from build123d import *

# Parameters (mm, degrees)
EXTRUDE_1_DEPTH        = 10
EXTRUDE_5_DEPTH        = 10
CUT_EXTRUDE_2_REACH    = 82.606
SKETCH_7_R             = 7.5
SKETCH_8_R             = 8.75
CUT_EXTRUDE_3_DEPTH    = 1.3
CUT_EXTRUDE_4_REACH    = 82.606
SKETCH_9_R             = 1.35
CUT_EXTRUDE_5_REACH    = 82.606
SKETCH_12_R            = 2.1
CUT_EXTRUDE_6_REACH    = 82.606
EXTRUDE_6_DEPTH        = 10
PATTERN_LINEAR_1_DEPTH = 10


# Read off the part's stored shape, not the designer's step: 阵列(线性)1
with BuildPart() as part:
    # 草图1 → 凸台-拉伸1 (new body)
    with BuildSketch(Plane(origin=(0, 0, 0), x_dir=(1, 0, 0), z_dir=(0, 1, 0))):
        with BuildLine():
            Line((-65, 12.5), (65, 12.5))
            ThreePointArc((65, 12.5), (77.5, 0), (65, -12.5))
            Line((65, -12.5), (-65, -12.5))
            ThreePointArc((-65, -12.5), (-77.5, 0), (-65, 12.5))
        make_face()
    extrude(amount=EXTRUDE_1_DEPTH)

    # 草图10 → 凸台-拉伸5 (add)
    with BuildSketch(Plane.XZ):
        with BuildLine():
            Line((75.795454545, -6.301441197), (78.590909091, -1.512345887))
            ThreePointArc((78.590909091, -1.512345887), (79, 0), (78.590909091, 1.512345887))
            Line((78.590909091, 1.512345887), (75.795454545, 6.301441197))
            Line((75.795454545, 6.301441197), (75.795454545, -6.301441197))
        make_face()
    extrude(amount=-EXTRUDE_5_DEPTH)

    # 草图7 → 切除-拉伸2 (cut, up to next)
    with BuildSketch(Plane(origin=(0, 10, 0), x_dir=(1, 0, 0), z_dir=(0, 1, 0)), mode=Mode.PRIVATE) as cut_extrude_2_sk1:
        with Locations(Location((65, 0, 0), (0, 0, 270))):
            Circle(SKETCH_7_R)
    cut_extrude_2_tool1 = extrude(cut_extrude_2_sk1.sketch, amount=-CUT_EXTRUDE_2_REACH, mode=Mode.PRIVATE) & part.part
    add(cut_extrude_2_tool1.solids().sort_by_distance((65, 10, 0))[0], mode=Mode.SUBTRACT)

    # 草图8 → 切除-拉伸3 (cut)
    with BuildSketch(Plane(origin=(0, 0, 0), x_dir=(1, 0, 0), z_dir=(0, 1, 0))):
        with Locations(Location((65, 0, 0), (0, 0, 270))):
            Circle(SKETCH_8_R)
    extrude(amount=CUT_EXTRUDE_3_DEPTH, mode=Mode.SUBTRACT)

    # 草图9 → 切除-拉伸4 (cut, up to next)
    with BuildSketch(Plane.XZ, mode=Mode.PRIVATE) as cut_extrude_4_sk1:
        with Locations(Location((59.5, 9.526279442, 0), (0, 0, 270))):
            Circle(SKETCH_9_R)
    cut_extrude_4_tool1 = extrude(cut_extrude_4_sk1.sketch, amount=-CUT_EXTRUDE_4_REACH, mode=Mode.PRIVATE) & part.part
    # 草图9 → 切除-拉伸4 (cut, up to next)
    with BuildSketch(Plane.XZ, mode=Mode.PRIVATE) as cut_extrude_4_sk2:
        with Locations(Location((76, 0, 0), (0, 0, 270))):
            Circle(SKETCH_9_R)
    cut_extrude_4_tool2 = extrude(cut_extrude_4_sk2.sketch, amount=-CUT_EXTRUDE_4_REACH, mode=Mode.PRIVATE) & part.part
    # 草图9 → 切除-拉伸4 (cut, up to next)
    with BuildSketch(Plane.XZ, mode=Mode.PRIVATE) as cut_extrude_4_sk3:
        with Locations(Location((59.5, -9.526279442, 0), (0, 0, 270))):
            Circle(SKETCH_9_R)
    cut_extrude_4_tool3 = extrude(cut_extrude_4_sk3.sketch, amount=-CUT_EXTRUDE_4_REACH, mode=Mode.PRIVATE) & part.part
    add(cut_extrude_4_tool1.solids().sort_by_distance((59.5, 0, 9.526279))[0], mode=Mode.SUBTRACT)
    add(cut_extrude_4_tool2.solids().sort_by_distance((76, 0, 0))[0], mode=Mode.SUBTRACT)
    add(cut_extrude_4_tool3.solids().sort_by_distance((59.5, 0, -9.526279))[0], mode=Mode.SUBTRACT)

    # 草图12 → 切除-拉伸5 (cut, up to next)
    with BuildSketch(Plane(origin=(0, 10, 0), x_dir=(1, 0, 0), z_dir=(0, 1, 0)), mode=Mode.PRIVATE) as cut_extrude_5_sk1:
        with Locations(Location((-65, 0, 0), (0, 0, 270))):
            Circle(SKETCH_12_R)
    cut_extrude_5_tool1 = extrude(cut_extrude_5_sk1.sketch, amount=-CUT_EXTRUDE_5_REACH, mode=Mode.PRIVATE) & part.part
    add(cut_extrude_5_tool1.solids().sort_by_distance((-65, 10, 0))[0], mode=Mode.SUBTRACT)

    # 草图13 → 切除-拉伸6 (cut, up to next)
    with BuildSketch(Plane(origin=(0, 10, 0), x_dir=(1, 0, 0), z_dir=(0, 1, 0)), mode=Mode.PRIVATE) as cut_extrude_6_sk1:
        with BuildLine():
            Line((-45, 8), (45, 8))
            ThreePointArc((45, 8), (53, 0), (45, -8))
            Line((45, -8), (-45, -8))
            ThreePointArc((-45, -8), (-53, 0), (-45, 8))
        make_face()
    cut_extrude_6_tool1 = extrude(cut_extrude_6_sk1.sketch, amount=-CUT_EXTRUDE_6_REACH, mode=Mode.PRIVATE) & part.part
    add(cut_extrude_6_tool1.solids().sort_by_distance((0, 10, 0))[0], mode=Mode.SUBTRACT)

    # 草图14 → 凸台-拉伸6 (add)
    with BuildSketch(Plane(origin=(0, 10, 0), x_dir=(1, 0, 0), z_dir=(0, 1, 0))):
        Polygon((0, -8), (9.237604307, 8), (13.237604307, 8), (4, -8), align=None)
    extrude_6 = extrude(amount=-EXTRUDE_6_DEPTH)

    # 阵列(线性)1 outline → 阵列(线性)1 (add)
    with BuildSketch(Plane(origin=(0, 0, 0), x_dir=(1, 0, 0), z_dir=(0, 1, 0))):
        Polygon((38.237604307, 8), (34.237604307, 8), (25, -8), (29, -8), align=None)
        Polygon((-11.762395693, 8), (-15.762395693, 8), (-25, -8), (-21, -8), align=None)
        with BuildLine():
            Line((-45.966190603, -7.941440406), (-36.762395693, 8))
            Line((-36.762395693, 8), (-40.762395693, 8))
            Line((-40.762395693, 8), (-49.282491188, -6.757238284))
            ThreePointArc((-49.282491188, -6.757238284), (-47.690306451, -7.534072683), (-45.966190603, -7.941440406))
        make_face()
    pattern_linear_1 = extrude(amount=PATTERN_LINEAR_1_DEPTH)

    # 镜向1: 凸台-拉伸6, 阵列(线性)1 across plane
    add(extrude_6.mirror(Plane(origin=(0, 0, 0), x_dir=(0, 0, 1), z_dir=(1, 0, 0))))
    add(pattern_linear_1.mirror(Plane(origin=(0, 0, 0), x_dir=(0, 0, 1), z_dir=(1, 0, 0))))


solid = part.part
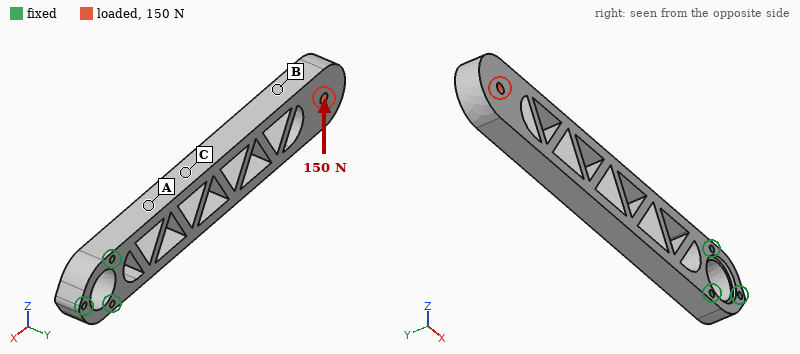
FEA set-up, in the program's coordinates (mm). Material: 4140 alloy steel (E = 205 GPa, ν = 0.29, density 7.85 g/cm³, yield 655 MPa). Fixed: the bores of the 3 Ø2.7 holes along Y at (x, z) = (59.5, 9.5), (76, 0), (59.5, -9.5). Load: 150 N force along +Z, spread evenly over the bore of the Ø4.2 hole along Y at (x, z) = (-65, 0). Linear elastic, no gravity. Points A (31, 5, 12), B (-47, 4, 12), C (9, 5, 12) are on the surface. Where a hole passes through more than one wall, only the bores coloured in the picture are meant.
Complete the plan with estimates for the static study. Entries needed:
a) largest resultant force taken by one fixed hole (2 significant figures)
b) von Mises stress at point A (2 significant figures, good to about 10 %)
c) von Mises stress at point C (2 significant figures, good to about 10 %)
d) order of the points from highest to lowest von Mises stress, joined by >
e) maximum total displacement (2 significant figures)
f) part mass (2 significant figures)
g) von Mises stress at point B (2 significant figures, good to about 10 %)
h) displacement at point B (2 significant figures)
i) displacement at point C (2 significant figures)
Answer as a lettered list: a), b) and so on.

a) 930 N
b) 19 MPa
c) 14 MPa
d) A > C > B
e) 59 µm
f) 190 g
g) 4.1 MPa
h) 42 µm
i) 13 µm
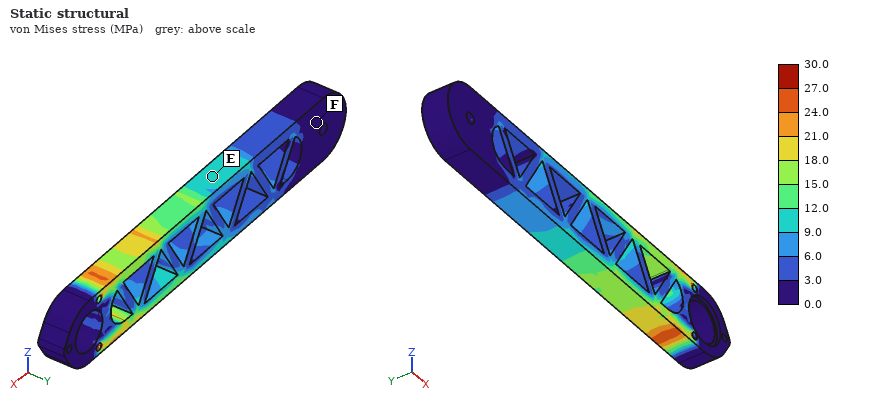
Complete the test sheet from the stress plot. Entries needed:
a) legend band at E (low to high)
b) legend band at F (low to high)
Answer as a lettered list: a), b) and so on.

a) 9.0 to 12.0 MPa
b) 0.0 to 3.0 MPa
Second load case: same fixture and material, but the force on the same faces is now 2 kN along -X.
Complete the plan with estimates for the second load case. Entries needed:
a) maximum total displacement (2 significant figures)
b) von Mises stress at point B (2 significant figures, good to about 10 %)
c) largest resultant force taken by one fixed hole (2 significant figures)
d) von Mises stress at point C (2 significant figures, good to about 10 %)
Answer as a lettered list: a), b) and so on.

a) 12 µm
b) 17 MPa
c) 1000 N
d) 20 MPa
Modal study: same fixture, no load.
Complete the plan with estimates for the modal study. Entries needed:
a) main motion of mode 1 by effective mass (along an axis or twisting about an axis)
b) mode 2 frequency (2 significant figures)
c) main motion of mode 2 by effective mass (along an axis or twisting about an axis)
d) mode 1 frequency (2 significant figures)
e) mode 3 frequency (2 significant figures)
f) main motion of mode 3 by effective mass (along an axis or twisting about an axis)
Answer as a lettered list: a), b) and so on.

a) along Y
b) 1100 Hz
c) along Z
d) 340 Hz
e) 2300 Hz
f) along Y
